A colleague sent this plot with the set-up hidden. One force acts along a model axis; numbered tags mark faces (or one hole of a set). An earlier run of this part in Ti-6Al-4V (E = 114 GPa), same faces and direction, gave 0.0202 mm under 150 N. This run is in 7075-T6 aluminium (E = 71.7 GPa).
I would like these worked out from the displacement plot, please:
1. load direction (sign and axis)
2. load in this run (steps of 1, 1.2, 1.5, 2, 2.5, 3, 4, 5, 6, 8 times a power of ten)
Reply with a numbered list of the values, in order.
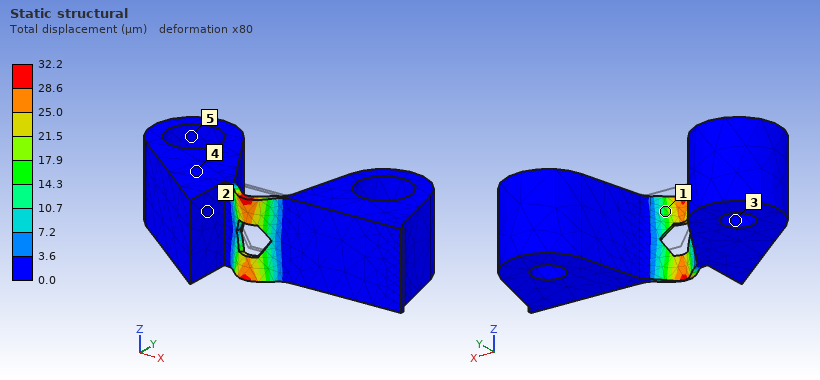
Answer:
1. -Y
2. 150 N
